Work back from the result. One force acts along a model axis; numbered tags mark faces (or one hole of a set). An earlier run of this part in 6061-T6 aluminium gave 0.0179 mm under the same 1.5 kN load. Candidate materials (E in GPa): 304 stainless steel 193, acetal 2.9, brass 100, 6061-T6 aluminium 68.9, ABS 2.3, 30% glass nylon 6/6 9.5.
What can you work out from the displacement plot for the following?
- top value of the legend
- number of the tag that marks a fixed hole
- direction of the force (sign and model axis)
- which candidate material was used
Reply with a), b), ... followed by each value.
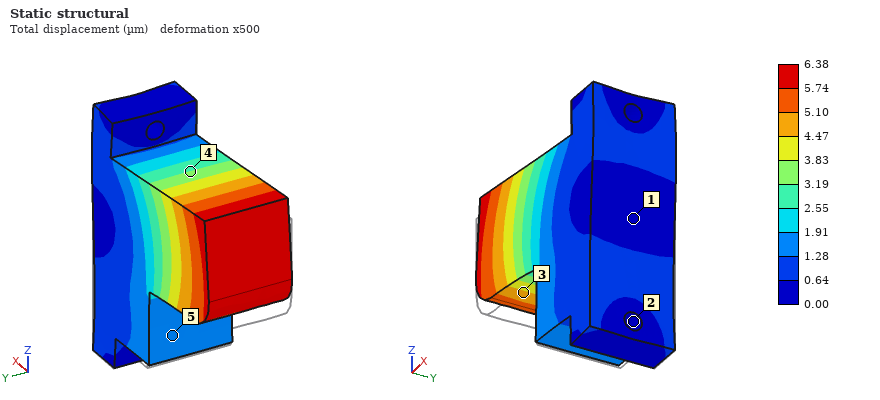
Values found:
a) 6.38 µm
b) 2
c) +Z
d) 304 stainless steel
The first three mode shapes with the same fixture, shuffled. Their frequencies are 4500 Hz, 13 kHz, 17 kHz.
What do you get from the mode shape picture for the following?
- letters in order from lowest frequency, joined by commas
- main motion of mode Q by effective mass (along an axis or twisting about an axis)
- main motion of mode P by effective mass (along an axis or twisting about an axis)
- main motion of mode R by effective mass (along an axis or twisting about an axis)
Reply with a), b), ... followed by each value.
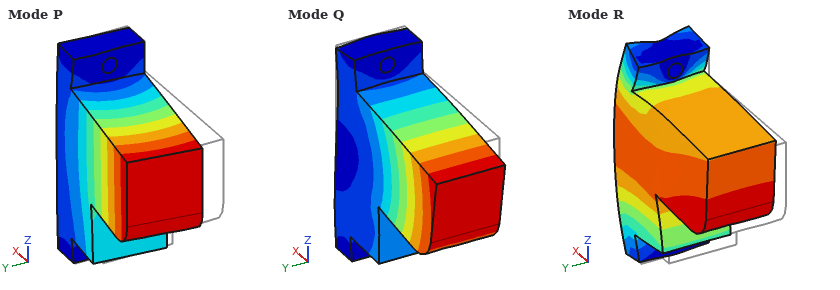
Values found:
a) P, Q, R
b) along Z
c) along Y
d) along X
